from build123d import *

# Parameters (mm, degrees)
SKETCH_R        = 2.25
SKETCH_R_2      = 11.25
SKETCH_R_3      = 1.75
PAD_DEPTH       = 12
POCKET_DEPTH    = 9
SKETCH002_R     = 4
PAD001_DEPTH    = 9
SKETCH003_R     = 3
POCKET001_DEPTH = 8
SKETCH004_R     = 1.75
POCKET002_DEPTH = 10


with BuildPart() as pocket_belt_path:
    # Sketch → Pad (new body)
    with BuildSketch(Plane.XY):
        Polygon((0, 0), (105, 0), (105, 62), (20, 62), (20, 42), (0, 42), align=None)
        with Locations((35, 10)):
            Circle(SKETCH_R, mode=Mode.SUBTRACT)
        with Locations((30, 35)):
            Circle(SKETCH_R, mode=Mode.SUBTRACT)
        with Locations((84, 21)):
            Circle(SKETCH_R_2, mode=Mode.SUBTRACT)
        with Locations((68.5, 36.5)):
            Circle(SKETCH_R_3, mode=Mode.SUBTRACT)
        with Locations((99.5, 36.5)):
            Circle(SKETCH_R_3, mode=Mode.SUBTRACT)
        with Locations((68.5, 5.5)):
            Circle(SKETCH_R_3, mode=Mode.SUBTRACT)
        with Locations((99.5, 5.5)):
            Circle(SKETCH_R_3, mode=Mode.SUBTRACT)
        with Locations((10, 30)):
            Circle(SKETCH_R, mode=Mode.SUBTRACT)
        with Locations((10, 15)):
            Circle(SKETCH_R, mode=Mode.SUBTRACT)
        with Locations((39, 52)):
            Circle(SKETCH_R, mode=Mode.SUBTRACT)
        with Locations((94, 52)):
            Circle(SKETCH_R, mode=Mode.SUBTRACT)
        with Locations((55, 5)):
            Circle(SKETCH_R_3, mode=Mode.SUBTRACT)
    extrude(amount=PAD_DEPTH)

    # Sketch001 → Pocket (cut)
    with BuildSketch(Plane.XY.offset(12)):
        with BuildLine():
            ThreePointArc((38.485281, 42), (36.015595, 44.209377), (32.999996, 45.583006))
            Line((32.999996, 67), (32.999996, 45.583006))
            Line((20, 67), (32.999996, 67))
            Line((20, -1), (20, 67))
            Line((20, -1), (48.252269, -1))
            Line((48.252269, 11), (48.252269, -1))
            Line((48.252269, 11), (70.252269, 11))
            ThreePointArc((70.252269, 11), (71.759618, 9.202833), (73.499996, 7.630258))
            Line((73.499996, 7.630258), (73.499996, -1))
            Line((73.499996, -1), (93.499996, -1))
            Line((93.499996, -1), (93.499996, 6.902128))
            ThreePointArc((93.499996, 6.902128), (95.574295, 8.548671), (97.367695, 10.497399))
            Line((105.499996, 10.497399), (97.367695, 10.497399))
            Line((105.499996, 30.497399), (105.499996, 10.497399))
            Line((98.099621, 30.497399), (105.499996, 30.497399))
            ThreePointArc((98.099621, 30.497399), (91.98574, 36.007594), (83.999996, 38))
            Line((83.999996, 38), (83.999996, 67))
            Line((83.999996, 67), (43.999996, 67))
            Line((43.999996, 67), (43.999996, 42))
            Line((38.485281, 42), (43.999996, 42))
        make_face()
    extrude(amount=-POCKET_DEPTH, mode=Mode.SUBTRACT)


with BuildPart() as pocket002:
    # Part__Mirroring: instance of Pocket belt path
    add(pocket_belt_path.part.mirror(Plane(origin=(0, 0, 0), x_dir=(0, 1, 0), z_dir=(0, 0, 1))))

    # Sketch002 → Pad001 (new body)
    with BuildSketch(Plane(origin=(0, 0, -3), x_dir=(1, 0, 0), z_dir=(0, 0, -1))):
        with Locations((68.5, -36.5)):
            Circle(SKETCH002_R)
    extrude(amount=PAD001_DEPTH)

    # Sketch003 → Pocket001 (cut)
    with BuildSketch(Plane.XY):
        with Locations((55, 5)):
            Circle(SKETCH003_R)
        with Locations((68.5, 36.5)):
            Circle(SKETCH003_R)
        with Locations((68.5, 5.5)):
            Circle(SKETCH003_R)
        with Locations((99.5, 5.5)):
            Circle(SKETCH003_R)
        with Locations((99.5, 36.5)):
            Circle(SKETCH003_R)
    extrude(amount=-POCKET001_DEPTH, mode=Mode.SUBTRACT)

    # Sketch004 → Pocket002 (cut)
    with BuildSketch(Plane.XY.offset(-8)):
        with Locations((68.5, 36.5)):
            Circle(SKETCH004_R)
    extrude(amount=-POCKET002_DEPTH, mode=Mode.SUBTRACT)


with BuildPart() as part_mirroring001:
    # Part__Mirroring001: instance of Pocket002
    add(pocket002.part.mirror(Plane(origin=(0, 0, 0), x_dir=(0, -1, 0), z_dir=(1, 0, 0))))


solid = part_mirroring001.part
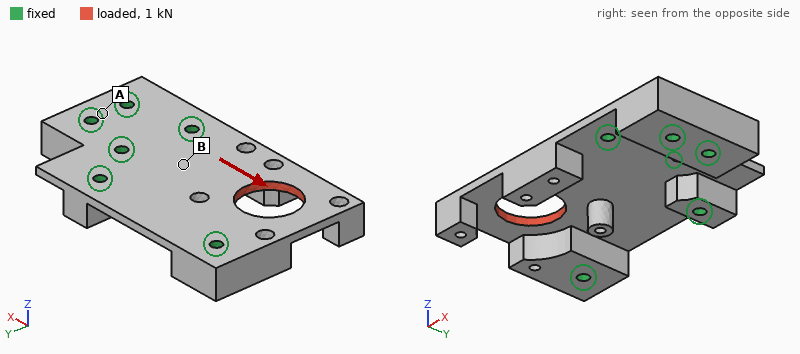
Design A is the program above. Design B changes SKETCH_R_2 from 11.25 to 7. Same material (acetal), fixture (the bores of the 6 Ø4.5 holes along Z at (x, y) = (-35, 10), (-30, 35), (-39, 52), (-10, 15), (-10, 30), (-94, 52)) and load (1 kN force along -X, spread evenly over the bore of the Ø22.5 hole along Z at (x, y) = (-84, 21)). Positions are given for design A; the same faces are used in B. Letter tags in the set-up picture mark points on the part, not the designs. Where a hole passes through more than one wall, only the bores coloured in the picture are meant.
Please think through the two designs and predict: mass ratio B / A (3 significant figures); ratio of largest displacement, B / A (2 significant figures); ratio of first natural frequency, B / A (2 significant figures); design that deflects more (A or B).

1.02
0.77
1.1
A
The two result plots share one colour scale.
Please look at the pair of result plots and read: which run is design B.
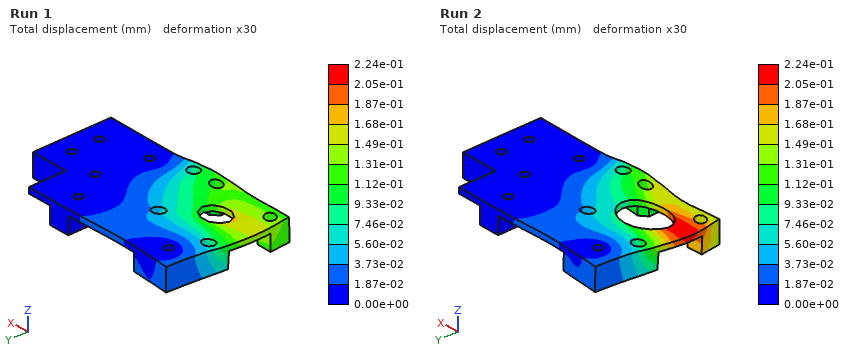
Run 1
